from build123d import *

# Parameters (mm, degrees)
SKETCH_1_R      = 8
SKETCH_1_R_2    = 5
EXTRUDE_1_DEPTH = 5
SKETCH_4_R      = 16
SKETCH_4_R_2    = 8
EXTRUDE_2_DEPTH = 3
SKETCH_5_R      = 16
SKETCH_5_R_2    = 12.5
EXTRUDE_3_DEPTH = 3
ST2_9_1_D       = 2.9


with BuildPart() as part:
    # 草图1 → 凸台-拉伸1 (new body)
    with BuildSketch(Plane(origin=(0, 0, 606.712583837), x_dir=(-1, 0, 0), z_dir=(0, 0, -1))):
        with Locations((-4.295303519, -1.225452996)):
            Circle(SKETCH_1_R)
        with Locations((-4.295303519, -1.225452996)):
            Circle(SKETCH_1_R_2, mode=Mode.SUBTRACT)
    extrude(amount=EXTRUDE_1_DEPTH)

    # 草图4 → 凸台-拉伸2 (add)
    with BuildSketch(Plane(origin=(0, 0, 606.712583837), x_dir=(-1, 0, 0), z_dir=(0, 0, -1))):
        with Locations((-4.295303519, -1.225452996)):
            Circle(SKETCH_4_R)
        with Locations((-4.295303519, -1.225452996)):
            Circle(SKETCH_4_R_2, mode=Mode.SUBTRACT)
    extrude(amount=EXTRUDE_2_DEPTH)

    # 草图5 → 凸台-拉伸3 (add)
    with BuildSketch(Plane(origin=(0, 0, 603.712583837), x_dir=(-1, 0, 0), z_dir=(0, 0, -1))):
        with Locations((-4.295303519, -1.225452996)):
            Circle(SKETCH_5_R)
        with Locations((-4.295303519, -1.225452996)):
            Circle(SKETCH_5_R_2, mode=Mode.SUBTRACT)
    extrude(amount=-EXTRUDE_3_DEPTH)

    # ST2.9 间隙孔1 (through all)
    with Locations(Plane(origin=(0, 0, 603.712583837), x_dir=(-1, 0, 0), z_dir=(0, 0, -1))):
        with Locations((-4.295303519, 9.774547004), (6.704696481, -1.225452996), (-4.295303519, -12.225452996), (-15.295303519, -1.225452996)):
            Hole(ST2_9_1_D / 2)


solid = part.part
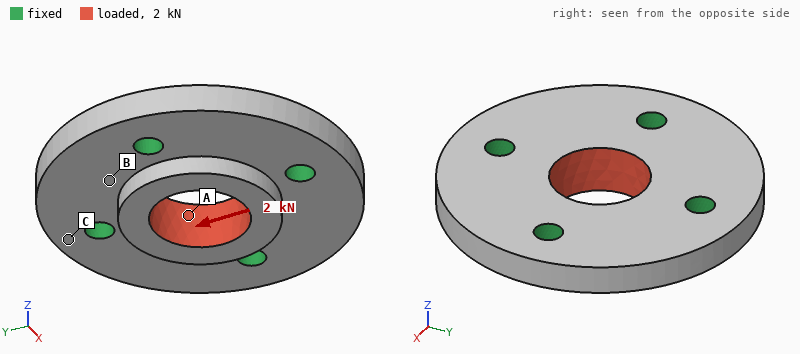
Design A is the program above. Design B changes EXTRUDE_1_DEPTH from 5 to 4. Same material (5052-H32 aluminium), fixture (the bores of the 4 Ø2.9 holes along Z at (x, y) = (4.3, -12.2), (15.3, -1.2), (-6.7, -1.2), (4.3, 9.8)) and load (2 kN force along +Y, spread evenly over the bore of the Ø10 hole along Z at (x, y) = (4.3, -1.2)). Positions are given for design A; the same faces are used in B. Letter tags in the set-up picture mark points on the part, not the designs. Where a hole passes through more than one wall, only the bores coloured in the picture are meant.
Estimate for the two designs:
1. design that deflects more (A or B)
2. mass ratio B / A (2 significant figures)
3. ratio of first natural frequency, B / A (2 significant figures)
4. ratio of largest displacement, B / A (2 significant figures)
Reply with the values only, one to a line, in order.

A
0.95
0.99
0.87
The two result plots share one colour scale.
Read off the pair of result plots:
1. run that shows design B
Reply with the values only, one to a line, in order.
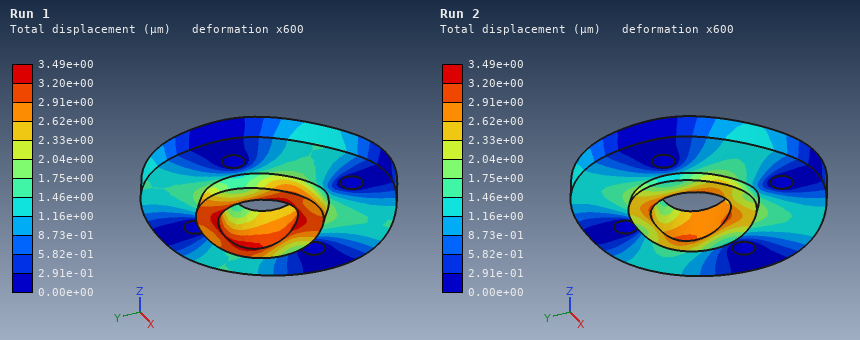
Run 2
